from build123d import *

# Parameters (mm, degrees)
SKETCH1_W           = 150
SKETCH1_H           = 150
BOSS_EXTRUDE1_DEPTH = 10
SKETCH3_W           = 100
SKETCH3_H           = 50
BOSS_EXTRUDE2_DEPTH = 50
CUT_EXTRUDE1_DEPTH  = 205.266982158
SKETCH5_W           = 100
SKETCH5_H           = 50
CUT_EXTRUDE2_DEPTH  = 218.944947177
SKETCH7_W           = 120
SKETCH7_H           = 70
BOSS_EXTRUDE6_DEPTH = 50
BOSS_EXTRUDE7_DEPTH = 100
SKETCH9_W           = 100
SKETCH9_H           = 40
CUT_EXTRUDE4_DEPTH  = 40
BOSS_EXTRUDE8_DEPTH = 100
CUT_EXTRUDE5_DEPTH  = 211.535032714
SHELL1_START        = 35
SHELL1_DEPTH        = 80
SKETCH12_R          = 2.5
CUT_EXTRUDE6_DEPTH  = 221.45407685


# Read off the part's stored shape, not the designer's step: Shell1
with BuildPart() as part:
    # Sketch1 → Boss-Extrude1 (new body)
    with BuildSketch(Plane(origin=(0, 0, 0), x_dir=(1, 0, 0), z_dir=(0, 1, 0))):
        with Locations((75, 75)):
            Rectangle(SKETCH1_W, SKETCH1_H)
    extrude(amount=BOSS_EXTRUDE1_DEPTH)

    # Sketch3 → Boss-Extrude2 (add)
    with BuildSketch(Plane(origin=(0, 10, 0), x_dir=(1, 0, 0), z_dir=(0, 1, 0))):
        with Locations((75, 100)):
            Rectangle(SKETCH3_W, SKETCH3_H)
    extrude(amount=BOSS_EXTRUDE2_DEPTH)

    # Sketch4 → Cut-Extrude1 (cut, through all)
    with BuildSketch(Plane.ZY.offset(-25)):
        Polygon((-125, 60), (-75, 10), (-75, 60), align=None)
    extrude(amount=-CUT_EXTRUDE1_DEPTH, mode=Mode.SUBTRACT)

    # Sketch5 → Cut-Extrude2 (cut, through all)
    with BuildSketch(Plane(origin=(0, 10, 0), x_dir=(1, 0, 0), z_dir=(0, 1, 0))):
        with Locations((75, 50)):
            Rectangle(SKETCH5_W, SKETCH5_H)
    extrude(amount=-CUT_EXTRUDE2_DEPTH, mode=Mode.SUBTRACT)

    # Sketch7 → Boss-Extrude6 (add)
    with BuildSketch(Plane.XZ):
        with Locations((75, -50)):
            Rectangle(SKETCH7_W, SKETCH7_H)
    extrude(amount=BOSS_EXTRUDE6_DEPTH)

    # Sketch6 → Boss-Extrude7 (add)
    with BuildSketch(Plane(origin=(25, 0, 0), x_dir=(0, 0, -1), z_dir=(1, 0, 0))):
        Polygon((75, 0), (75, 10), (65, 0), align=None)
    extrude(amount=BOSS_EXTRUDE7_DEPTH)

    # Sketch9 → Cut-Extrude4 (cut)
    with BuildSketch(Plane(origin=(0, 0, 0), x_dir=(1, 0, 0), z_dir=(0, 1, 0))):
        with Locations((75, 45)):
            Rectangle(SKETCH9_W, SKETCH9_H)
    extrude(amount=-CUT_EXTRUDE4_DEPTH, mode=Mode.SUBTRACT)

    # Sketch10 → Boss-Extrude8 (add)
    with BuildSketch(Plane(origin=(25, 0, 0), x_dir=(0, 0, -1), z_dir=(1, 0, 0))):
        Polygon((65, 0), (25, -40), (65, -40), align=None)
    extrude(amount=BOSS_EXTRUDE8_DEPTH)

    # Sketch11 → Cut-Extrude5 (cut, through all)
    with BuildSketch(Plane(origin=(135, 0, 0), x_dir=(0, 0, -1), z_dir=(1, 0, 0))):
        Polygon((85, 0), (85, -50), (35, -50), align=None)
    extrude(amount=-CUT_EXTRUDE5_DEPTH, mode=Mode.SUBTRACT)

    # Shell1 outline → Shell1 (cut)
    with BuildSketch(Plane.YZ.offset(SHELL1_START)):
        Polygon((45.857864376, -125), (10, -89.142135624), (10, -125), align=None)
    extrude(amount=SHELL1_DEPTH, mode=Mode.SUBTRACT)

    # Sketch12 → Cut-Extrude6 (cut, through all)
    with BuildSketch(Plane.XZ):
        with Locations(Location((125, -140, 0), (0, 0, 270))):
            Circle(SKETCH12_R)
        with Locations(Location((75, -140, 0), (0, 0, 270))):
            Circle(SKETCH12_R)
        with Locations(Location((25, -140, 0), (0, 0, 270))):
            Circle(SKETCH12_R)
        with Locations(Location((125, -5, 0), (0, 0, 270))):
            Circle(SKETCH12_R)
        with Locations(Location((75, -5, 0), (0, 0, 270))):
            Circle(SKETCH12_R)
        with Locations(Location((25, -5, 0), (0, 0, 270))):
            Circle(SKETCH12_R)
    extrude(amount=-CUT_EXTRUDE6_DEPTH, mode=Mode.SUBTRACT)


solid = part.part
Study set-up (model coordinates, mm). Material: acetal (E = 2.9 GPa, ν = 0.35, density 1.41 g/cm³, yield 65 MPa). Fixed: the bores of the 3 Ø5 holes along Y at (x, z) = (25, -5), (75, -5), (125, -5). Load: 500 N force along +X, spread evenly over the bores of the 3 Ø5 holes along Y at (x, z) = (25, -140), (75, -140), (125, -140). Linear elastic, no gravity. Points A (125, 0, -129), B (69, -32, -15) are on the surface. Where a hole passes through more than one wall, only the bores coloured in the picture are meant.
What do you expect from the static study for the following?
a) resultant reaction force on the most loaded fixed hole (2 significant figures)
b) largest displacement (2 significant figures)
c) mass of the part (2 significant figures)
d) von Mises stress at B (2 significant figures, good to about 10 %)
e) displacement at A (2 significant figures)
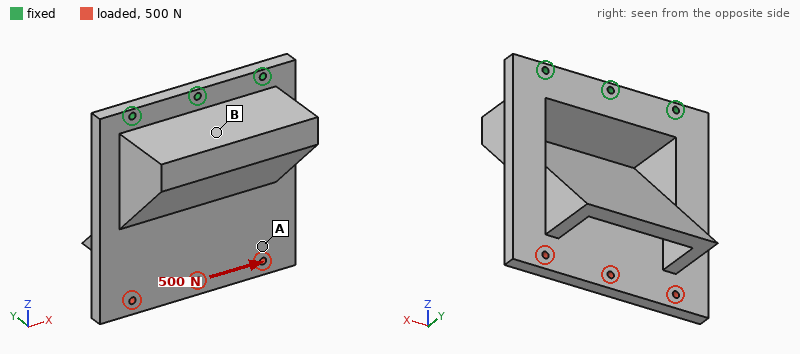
640 N
0.52 mm
620 g
1.3 MPa
0.37 mm
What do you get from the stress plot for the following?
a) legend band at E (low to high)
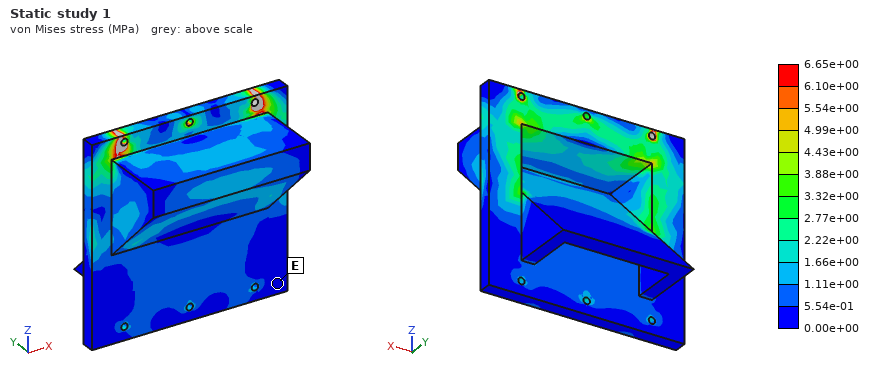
0.00e+00 to 5.54e-01 MPa
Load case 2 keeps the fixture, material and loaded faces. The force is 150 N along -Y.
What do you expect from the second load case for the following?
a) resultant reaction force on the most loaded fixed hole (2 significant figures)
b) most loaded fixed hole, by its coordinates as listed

190 N
(75, -5)
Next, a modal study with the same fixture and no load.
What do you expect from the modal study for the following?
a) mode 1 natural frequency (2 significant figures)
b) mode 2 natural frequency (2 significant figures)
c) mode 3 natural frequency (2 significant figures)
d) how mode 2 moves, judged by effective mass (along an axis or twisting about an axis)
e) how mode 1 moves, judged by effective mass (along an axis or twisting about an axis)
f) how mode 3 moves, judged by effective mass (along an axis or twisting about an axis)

90 Hz
290 Hz
580 Hz
along X
along Y
along X
